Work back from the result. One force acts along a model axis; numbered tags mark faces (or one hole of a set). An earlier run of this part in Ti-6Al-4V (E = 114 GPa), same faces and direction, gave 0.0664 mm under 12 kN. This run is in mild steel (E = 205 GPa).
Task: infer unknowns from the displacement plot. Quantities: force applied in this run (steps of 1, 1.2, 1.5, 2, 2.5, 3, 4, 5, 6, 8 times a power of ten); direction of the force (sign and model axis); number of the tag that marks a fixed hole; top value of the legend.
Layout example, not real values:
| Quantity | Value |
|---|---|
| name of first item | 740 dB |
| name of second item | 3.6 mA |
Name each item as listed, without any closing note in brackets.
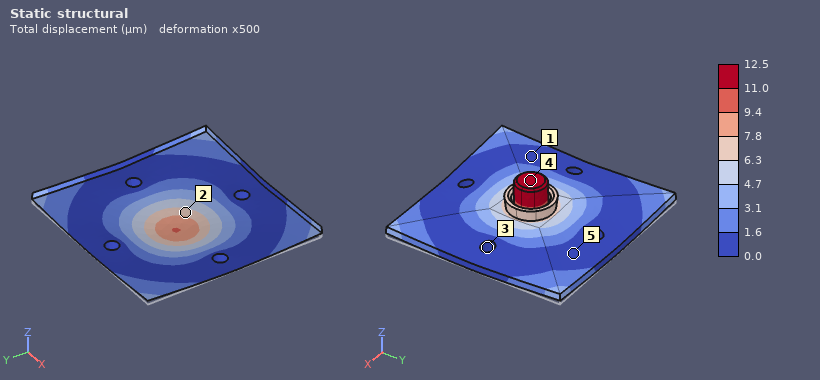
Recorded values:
| Quantity | Value |
|---|---|
| force applied in this run | 4 kN |
| direction of the force | -Z |
| number of the tag that marks a fixed hole | 3 |
| top value of the legend | 12.5 µm |
